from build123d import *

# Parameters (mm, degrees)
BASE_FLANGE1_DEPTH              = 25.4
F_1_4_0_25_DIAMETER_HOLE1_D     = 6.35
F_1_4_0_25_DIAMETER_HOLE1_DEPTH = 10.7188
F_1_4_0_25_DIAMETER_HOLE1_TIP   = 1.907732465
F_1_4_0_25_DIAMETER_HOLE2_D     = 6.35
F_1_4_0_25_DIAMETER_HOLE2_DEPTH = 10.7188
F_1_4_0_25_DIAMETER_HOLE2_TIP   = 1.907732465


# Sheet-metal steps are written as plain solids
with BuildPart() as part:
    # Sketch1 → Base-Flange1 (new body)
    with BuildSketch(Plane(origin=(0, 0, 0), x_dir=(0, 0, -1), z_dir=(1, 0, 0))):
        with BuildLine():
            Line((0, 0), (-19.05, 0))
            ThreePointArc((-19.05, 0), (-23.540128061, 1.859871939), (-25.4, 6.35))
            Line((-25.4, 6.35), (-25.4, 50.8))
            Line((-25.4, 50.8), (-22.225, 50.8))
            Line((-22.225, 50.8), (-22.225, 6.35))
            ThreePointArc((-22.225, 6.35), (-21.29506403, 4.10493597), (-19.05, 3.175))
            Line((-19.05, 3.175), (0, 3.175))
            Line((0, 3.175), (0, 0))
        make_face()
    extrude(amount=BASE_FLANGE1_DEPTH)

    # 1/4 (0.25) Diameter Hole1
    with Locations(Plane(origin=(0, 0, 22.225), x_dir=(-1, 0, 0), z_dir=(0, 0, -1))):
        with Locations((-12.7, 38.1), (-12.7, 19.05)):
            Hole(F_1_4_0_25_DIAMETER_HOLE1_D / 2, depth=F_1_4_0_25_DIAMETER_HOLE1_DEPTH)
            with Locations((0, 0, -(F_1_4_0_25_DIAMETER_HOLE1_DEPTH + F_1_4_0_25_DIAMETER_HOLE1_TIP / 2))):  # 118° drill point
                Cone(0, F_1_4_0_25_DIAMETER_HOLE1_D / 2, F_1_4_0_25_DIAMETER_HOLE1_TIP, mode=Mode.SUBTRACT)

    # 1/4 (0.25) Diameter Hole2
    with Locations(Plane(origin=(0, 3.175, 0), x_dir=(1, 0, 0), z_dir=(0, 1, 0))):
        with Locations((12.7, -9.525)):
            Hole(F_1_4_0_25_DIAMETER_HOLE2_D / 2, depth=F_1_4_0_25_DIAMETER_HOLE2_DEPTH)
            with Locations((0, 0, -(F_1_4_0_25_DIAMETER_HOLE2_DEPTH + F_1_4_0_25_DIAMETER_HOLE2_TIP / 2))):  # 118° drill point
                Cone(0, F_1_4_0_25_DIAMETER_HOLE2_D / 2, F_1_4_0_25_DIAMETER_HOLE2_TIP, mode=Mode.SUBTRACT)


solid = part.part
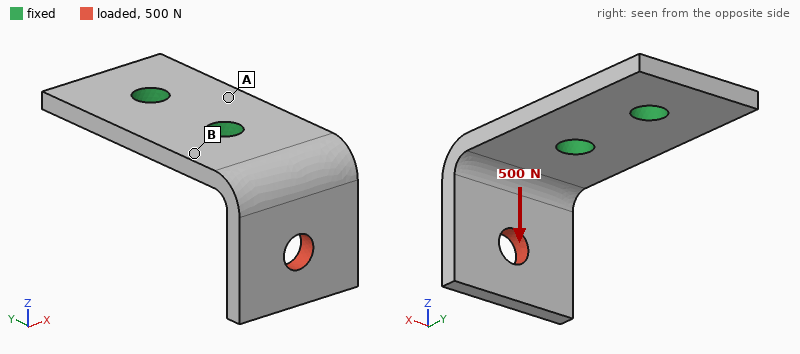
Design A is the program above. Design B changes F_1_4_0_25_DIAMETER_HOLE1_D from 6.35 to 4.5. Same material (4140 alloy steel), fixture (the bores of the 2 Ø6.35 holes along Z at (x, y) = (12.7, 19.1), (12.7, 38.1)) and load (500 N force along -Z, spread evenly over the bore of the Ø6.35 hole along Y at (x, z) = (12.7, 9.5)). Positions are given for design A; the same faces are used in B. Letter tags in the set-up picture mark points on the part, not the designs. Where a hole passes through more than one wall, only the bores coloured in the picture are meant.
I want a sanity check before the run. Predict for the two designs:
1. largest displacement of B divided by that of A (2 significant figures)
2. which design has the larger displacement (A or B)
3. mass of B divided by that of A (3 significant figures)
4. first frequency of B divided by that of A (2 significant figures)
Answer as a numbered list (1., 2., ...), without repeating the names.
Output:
1. 1.2
2. B
3. 1.02
4. 0.95
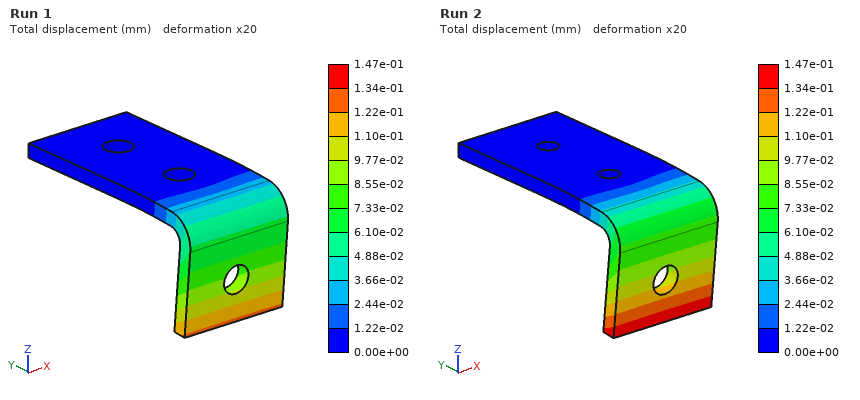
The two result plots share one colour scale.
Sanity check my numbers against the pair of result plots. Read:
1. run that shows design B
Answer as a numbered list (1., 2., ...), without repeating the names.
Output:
1. Run 2
